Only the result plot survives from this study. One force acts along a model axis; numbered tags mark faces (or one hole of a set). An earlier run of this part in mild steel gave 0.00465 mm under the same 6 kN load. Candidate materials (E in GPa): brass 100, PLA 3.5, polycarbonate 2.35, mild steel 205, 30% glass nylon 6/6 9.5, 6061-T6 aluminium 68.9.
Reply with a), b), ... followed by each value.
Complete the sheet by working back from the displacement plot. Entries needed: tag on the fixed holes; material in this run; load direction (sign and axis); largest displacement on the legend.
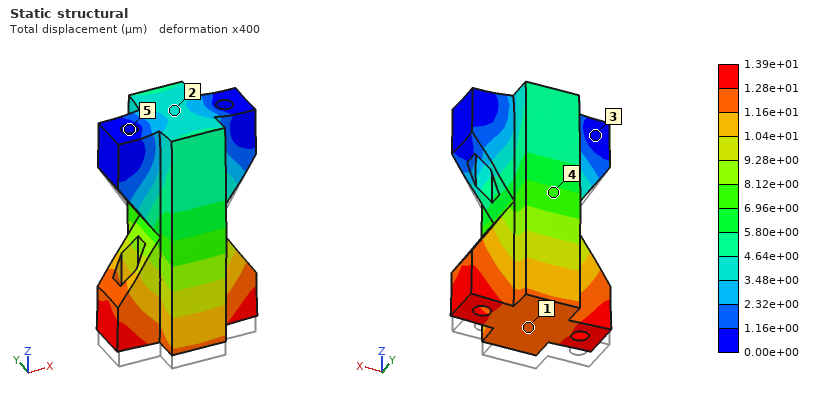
a) 5
b) 6061-T6 aluminium
c) +Z
d) 1.39e+01 µm
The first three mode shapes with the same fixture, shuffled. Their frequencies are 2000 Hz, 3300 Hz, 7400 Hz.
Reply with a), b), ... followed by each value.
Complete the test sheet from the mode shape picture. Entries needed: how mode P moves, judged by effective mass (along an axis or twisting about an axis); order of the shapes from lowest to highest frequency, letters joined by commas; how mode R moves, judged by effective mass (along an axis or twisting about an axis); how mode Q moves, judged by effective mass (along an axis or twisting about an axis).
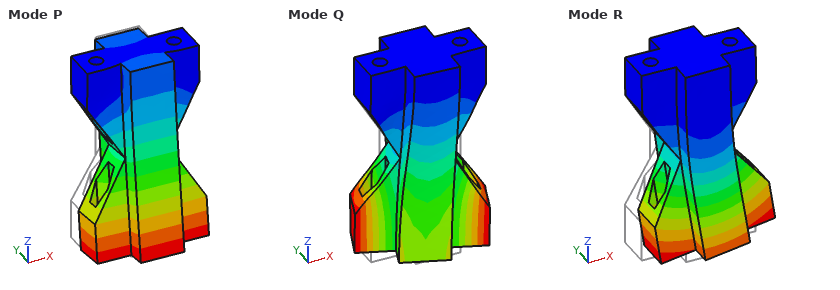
a) along Y
b) P, R, Q
c) along X
d) twisting about Z
